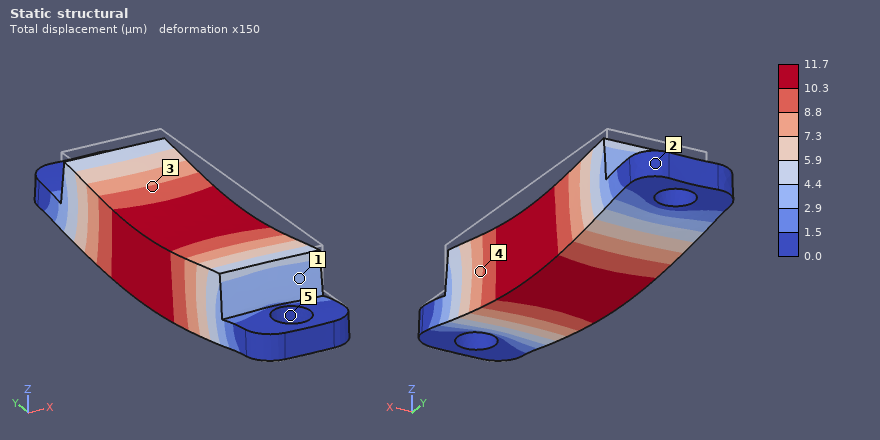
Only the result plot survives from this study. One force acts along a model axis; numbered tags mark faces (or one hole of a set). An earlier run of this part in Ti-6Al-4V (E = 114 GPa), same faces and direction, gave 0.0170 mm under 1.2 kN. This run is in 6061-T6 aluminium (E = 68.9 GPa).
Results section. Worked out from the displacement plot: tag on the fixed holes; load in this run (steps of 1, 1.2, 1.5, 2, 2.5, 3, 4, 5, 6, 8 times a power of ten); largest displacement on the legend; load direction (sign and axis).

5
500 N
11.7 µm
-Z
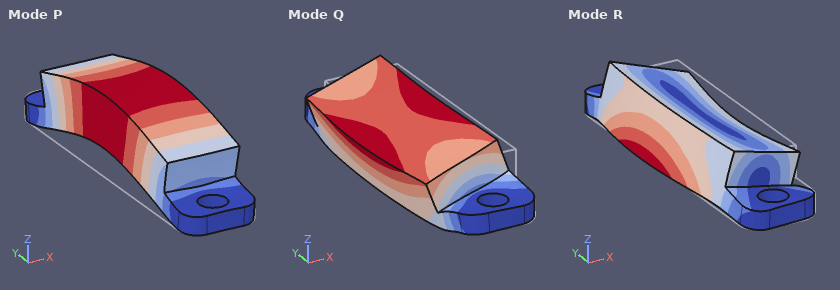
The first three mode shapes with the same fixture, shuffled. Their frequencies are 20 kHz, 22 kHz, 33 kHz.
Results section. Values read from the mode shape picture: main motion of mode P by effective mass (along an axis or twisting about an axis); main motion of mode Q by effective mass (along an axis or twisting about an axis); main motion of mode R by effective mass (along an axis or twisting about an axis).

along Z
along X
along X
